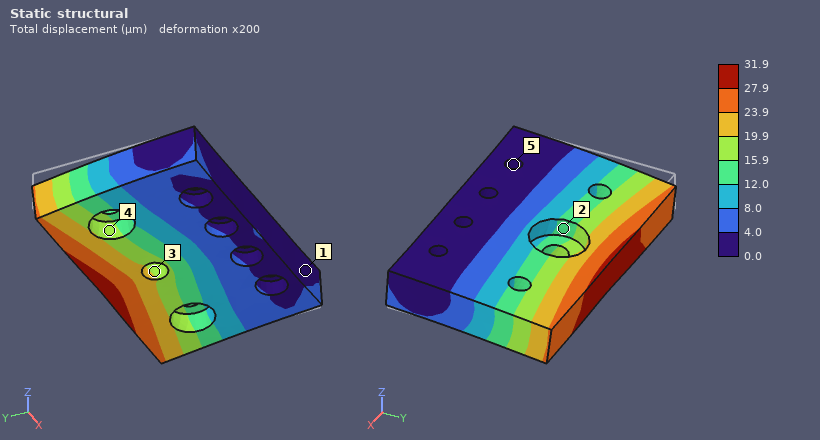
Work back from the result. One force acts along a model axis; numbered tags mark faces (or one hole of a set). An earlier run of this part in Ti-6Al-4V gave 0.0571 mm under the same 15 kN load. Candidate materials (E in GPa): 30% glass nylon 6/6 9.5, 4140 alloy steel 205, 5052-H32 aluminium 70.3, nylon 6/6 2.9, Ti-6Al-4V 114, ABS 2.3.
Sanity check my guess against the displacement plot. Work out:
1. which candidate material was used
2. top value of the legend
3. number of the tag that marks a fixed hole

4140 alloy steel
31.9 µm
5
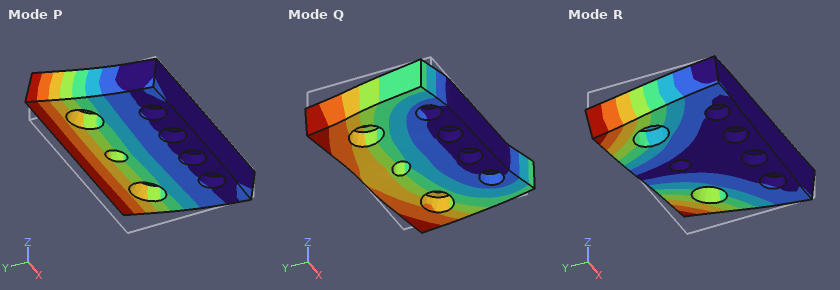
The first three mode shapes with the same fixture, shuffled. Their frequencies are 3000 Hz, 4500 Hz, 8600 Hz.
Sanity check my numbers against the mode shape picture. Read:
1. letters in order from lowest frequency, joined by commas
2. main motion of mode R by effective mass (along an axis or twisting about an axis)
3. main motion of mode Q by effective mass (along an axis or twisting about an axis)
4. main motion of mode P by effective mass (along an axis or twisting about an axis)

P, R, Q
twisting about Y
along X
along Z
